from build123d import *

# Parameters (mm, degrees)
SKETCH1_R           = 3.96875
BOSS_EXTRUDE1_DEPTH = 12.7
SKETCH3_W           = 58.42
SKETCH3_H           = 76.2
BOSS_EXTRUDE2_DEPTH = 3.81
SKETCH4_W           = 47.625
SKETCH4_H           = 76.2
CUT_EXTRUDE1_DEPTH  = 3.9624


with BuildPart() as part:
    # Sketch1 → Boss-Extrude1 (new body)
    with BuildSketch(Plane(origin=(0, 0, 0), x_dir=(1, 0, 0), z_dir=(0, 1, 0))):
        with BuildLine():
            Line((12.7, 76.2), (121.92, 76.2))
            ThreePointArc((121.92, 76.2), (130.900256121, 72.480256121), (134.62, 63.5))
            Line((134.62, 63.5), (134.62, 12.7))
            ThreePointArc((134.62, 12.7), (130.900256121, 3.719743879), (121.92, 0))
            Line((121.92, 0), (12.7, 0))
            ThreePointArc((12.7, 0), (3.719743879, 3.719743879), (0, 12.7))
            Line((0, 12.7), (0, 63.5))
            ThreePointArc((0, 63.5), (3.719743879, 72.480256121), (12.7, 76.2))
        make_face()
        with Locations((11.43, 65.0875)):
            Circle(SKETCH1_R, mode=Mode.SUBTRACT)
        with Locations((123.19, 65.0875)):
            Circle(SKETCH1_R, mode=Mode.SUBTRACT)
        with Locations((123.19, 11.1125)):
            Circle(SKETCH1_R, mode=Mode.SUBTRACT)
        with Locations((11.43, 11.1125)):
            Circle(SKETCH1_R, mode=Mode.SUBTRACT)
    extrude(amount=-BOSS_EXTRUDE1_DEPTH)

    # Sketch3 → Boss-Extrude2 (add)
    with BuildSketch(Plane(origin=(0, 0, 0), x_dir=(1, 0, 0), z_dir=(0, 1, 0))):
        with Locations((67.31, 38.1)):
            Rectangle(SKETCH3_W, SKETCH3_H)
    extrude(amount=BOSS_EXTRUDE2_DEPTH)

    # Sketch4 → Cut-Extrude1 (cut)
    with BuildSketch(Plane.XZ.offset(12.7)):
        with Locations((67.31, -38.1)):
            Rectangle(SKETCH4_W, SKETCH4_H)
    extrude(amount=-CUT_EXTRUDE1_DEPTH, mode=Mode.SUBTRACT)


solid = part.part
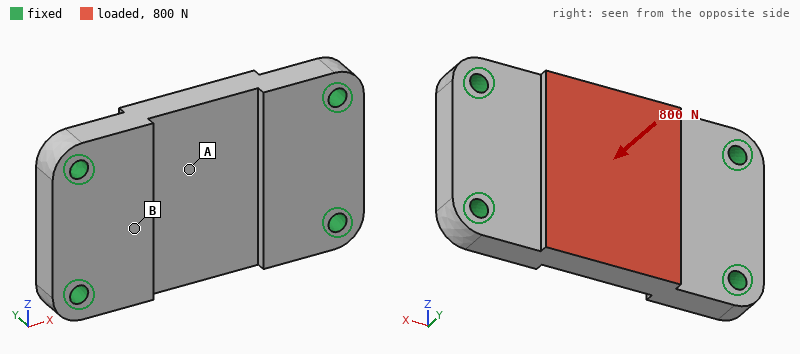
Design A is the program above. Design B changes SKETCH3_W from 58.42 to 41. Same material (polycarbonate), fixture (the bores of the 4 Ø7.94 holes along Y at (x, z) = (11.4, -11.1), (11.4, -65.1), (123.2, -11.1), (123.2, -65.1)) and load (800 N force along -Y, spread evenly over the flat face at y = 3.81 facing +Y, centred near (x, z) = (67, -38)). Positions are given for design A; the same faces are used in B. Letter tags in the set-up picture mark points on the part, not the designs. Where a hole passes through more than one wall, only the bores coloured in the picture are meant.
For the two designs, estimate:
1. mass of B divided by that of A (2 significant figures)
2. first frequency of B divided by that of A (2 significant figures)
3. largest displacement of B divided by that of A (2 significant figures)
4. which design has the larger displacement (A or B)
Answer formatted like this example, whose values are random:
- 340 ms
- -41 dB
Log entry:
- 0.96
- 0.98
- 1.2
- B
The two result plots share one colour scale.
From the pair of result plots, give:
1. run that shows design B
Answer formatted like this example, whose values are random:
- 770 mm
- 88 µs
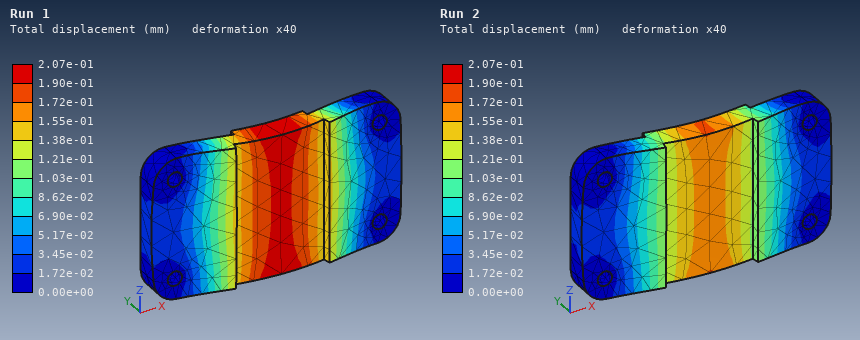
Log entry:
- Run 1
